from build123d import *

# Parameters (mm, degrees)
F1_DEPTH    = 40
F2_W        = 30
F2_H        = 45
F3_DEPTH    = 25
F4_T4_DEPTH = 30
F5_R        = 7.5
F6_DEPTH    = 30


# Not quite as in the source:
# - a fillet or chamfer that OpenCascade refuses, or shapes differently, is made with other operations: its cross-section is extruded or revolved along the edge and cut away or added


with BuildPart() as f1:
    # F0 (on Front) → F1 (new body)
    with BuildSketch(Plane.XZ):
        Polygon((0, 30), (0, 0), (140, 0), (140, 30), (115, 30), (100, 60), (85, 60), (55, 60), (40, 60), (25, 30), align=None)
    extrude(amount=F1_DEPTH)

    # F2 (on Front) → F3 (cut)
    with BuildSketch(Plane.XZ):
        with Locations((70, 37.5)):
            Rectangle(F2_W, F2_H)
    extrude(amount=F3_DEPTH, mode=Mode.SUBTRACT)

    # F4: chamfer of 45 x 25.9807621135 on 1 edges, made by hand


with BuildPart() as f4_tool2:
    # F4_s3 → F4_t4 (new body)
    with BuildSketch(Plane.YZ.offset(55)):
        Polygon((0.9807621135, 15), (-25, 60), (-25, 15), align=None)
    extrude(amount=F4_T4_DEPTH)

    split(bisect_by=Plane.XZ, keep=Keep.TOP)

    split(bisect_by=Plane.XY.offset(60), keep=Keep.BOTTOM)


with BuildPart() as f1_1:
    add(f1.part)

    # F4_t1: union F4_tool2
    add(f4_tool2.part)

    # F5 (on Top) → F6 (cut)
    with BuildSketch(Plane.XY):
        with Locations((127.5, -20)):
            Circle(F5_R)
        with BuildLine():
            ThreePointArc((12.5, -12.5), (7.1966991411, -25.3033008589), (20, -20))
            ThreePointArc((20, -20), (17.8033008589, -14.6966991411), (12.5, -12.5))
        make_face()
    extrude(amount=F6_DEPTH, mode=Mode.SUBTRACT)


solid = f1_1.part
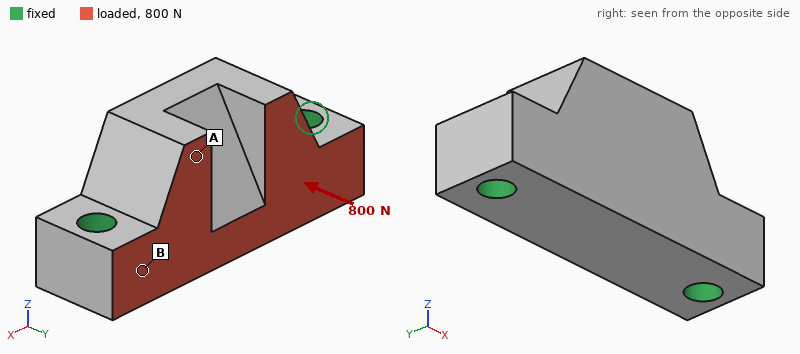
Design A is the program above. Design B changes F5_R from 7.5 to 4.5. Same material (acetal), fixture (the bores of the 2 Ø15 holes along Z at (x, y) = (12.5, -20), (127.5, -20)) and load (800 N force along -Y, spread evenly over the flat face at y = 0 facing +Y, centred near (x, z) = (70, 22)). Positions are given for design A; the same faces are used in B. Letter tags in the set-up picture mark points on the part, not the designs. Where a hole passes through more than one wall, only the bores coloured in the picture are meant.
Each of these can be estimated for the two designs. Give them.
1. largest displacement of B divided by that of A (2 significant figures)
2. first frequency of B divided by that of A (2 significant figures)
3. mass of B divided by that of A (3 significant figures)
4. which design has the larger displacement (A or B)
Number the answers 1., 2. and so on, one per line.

1. 1.2
2. 0.93
3. 1.01
4. B
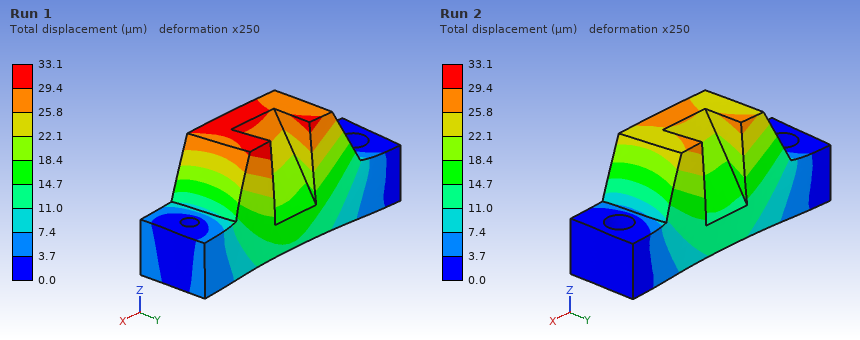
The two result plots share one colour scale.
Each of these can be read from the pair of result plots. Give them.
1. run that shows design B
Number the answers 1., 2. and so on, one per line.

1. Run 1
